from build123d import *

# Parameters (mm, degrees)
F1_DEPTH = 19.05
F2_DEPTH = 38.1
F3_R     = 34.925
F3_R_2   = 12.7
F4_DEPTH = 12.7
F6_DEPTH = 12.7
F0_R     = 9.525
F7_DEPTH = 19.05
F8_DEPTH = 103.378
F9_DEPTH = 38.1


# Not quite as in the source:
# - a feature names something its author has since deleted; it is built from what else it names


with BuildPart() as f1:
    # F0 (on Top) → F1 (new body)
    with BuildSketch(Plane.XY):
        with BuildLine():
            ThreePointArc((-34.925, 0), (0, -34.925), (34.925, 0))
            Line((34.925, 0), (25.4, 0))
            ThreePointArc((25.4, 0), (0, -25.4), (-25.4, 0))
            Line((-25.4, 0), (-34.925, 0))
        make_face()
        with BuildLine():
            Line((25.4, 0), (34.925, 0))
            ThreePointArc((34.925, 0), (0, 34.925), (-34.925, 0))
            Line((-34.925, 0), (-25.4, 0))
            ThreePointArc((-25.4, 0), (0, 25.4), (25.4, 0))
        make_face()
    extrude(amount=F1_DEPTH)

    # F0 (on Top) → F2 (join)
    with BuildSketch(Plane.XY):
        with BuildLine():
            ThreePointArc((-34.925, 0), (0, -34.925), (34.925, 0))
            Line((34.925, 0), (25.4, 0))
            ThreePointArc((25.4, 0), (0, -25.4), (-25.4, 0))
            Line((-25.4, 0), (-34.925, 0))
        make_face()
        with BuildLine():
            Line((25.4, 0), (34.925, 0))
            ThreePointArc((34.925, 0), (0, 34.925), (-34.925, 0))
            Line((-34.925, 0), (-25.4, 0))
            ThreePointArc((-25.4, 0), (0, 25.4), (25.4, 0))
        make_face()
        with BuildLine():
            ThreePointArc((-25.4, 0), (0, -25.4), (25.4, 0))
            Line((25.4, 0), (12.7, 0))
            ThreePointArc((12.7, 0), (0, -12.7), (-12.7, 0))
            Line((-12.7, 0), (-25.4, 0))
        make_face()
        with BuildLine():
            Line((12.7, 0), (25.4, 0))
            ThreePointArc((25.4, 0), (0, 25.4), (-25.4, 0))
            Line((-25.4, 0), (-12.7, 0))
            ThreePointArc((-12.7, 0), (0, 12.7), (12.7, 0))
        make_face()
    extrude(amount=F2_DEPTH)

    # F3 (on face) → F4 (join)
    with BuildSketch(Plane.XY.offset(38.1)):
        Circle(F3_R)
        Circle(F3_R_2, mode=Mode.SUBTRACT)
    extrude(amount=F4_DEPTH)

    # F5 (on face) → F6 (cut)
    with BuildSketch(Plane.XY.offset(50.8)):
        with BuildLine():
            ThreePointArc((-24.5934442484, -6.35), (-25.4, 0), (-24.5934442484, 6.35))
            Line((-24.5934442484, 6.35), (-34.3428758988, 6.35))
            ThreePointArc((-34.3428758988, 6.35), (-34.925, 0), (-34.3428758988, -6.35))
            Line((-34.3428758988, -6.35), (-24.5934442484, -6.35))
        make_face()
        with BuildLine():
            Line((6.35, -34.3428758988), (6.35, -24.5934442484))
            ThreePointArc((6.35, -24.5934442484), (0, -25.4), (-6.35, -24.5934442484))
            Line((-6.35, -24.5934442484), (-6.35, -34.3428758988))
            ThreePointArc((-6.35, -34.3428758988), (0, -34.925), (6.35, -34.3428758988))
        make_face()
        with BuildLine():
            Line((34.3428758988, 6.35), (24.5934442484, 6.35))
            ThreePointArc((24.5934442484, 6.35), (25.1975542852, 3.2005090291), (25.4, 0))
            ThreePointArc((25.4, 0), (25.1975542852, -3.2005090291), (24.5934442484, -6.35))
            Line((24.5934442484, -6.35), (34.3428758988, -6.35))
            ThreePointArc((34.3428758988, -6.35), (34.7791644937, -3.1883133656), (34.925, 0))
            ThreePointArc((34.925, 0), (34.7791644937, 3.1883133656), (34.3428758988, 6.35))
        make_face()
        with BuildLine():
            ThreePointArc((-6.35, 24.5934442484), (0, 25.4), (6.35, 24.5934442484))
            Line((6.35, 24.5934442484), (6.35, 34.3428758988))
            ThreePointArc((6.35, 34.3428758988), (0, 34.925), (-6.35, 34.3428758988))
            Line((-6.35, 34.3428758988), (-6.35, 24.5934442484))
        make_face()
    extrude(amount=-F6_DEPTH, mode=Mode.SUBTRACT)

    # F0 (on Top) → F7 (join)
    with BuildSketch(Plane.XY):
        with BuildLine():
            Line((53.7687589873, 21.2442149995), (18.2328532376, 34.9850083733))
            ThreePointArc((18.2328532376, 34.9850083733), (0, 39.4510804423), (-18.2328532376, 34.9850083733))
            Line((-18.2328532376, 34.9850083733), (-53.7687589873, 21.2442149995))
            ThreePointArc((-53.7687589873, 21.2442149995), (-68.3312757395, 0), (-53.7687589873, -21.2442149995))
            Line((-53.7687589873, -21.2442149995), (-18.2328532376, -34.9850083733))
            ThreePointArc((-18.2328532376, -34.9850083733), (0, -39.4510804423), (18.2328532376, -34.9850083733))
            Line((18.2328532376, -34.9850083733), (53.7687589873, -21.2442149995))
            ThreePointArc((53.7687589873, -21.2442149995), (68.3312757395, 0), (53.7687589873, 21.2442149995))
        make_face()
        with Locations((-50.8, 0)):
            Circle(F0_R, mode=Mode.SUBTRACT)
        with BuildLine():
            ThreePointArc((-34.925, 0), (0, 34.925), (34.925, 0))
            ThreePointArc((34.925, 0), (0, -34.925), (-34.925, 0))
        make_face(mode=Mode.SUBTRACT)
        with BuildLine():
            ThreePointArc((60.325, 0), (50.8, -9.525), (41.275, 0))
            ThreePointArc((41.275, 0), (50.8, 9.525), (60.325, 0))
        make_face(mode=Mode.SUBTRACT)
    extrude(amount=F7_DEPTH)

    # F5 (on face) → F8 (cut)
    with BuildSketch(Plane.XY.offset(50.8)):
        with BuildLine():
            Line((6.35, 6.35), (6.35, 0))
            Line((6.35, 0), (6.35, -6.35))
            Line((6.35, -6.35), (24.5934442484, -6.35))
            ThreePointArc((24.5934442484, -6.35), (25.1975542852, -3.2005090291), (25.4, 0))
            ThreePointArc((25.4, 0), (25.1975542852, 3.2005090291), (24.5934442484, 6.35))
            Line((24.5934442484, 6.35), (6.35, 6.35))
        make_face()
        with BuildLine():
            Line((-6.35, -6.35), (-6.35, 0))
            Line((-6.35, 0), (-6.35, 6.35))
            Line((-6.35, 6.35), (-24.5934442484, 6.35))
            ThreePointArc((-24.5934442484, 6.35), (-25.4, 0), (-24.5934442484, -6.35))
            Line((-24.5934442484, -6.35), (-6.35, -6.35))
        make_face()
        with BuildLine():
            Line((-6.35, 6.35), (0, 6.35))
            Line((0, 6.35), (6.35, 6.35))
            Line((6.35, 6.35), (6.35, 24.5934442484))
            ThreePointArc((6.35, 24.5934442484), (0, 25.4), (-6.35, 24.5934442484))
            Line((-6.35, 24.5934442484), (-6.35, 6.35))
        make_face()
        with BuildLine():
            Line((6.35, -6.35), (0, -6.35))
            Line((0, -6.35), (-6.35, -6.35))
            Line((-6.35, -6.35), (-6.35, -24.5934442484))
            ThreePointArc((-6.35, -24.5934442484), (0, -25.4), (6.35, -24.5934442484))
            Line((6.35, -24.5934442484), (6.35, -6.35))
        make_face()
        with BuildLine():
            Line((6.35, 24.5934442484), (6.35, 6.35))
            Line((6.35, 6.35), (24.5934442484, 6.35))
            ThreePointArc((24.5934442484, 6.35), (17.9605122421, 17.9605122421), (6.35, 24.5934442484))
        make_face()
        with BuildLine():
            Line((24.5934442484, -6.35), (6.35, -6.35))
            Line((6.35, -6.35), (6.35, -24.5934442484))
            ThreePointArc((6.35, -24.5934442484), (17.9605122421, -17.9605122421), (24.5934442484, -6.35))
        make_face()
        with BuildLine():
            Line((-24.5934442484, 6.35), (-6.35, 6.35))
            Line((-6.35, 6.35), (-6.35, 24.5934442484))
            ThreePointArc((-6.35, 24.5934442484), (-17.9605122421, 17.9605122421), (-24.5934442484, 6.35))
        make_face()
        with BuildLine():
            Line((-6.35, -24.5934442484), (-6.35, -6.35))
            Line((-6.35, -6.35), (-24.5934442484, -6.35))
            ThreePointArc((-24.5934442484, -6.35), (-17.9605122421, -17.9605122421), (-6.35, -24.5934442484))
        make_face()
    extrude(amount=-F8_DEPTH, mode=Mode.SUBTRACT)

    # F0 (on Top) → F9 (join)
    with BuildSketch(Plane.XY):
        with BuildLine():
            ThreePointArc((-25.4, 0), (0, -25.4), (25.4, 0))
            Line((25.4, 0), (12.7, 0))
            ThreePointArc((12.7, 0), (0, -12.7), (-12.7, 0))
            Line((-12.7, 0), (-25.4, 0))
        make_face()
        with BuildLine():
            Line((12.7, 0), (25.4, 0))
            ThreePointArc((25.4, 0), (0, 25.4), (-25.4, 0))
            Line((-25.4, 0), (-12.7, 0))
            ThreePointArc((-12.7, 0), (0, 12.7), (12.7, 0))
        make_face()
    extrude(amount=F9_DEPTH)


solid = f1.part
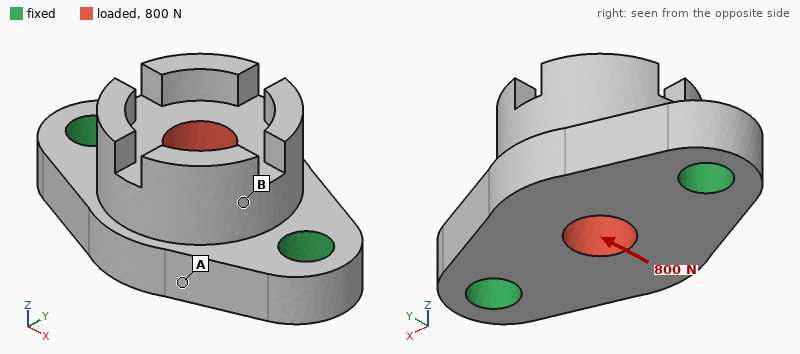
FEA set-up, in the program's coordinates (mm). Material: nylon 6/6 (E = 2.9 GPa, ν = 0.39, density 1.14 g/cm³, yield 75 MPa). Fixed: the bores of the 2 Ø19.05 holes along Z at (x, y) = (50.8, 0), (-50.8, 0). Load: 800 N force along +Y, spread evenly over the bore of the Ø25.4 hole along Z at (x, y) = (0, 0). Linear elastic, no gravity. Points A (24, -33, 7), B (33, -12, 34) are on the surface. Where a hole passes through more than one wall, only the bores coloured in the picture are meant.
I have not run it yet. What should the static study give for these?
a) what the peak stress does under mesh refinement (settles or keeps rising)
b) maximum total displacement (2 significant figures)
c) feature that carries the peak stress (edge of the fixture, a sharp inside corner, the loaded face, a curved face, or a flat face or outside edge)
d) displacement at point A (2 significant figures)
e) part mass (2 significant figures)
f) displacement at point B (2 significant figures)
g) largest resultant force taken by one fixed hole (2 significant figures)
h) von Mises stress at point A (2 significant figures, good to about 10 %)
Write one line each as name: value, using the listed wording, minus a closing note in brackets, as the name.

what the peak stress does under mesh refinement: keeps rising
maximum total displacement: 44 µm
feature that carries the peak stress: edge of the fixture
displacement at point A: 20 µm
part mass: 230 g
displacement at point B: 26 µm
largest resultant force taken by one fixed hole: 400 N
von Mises stress at point A: 0.70 MPa
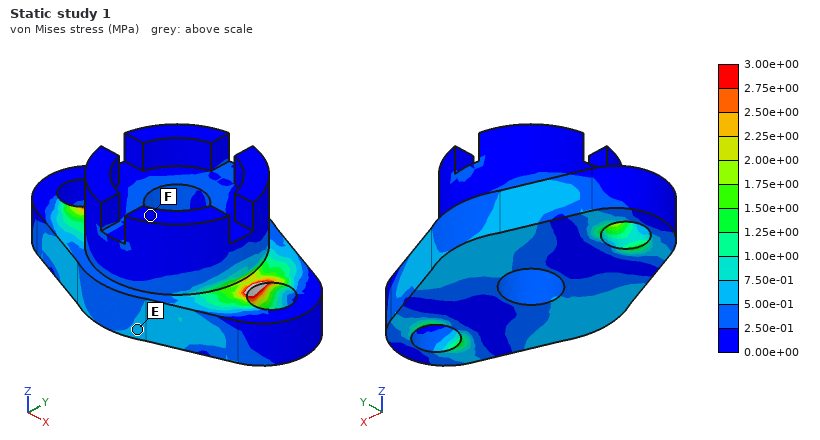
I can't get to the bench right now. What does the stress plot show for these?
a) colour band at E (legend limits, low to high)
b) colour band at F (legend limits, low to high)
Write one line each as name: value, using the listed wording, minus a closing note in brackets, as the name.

colour band at E: 5.00e-01 to 7.50e-01 MPa
colour band at F: 0.00e+00 to 2.50e-01 MPa
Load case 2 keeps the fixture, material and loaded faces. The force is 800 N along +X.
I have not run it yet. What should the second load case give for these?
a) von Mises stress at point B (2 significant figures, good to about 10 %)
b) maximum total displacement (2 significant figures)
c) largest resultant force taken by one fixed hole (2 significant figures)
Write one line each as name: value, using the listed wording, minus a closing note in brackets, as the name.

von Mises stress at point B: 0.13 MPa
maximum total displacement: 8.7 µm
largest resultant force taken by one fixed hole: 410 N
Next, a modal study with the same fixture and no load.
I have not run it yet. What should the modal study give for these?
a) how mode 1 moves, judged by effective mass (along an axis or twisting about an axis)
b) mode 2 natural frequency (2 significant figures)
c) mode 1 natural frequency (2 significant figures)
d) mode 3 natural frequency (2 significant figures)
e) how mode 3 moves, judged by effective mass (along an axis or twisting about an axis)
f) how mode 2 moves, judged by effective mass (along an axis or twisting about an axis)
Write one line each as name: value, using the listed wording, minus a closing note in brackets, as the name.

how mode 1 moves, judged by effective mass: along Y
mode 2 natural frequency: 2400 Hz
mode 1 natural frequency: 1500 Hz
mode 3 natural frequency: 3500 Hz
how mode 3 moves, judged by effective mass: along Y
how mode 2 moves, judged by effective mass: along Z
